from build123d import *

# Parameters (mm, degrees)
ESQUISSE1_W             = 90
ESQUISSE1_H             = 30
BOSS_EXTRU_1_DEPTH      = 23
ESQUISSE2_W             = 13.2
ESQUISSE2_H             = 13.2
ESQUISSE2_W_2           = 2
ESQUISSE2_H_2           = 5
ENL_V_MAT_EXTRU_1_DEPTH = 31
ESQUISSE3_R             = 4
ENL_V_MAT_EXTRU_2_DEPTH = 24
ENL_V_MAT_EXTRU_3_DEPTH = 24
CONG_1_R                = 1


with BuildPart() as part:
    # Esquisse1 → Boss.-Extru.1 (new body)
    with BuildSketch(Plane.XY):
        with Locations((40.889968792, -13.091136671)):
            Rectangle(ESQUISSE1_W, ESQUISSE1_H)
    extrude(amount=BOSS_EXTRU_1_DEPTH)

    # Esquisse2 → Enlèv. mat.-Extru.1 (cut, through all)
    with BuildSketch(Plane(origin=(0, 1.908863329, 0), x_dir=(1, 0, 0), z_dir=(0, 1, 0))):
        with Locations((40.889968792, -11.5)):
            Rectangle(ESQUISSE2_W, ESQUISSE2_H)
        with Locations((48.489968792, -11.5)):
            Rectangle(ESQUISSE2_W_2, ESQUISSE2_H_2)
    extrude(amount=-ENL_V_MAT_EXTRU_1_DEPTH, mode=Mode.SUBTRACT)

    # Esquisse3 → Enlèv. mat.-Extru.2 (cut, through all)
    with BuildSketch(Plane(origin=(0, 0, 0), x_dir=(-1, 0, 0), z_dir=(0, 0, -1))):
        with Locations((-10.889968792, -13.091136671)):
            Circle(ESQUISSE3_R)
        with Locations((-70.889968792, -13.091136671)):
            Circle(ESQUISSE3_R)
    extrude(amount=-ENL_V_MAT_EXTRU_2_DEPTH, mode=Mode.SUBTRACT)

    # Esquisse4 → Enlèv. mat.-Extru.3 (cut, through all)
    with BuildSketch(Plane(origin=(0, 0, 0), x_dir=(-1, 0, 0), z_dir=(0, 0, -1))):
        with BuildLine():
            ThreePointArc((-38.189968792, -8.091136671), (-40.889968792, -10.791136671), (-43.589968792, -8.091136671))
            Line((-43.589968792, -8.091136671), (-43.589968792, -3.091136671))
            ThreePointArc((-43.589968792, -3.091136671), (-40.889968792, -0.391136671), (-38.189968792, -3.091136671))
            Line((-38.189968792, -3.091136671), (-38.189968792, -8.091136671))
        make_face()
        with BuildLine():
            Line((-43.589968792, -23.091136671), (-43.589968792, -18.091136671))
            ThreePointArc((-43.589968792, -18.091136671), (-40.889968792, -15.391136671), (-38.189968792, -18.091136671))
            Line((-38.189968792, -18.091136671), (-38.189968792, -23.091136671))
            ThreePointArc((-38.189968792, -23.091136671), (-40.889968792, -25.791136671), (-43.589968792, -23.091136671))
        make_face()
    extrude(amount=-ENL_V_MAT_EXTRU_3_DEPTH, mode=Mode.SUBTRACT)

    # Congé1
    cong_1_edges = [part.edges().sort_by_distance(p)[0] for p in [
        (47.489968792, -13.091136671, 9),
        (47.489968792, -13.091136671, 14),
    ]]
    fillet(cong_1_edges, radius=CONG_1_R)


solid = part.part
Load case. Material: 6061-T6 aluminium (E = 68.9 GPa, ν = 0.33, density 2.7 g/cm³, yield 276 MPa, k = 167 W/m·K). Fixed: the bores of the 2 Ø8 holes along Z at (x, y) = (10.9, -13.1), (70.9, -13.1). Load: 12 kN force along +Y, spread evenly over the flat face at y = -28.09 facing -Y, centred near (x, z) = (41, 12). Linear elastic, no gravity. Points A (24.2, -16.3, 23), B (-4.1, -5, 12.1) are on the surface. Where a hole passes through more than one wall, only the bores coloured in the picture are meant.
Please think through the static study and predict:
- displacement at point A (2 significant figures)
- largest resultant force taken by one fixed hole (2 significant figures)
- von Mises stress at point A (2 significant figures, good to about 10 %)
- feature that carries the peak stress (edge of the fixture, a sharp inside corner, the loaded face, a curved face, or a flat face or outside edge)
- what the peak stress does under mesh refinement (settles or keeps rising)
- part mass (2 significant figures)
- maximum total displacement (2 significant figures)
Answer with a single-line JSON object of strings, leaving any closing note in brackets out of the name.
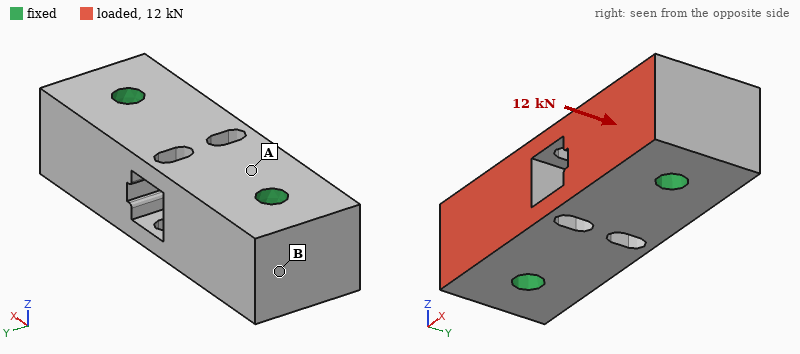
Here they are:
{"displacement at point A": "4.2 µm", "largest resultant force taken by one fixed hole": "6.0 kN", "von Mises stress at point A": "7.7 MPa", "feature that carries the peak stress": "a sharp inside corner", "what the peak stress does under mesh refinement": "keeps rising", "part mass": "140 g", "maximum total displacement": "8.4 µm"}
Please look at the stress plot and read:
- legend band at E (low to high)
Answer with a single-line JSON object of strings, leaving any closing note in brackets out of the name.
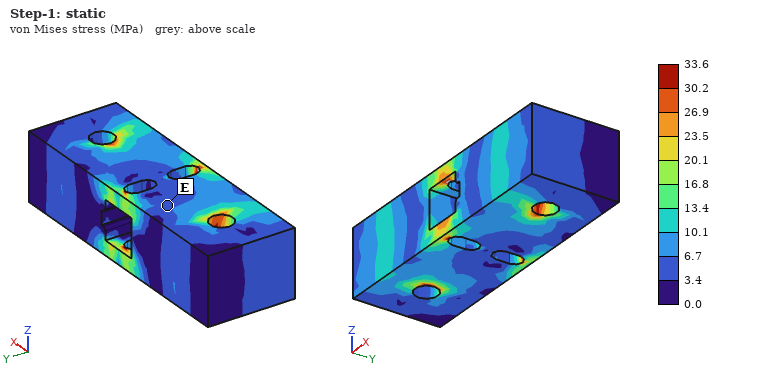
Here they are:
{"legend band at E": "3.4 to 6.7 MPa"}
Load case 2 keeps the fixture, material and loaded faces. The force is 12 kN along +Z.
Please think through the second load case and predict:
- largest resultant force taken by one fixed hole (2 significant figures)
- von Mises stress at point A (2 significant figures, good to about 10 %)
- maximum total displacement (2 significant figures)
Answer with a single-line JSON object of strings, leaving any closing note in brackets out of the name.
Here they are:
{"largest resultant force taken by one fixed hole": "6.0 kN", "von Mises stress at point A": "15 MPa", "maximum total displacement": "25 µm"}
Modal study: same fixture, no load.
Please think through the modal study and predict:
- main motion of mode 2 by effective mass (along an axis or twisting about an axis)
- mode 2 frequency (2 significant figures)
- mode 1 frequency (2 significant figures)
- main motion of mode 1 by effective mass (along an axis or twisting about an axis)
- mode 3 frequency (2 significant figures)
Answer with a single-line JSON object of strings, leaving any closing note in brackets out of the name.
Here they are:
{"main motion of mode 2 by effective mass": "along Z", "mode 2 frequency": "21 kHz", "mode 1 frequency": "16 kHz", "main motion of mode 1 by effective mass": "along Y", "mode 3 frequency": "24 kHz"}
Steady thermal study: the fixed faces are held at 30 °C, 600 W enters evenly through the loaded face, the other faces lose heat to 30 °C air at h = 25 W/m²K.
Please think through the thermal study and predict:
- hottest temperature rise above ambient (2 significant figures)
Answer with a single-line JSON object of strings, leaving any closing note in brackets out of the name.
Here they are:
{"hottest temperature rise above ambient": "51 K"}
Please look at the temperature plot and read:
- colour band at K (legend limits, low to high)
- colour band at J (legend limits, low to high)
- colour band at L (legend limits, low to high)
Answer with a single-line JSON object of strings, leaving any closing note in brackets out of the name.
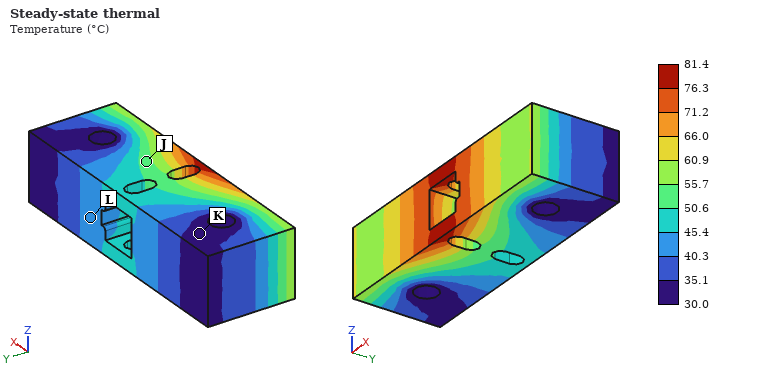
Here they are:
{"colour band at K": "30.0 to 35.1 °C", "colour band at J": "50.6 to 55.7 °C", "colour band at L": "40.3 to 45.4 °C"}
